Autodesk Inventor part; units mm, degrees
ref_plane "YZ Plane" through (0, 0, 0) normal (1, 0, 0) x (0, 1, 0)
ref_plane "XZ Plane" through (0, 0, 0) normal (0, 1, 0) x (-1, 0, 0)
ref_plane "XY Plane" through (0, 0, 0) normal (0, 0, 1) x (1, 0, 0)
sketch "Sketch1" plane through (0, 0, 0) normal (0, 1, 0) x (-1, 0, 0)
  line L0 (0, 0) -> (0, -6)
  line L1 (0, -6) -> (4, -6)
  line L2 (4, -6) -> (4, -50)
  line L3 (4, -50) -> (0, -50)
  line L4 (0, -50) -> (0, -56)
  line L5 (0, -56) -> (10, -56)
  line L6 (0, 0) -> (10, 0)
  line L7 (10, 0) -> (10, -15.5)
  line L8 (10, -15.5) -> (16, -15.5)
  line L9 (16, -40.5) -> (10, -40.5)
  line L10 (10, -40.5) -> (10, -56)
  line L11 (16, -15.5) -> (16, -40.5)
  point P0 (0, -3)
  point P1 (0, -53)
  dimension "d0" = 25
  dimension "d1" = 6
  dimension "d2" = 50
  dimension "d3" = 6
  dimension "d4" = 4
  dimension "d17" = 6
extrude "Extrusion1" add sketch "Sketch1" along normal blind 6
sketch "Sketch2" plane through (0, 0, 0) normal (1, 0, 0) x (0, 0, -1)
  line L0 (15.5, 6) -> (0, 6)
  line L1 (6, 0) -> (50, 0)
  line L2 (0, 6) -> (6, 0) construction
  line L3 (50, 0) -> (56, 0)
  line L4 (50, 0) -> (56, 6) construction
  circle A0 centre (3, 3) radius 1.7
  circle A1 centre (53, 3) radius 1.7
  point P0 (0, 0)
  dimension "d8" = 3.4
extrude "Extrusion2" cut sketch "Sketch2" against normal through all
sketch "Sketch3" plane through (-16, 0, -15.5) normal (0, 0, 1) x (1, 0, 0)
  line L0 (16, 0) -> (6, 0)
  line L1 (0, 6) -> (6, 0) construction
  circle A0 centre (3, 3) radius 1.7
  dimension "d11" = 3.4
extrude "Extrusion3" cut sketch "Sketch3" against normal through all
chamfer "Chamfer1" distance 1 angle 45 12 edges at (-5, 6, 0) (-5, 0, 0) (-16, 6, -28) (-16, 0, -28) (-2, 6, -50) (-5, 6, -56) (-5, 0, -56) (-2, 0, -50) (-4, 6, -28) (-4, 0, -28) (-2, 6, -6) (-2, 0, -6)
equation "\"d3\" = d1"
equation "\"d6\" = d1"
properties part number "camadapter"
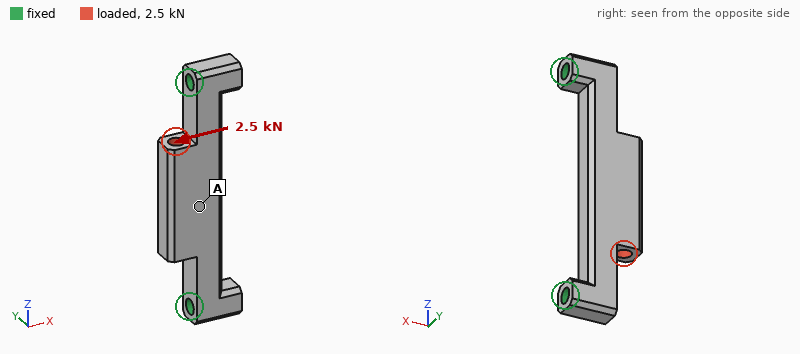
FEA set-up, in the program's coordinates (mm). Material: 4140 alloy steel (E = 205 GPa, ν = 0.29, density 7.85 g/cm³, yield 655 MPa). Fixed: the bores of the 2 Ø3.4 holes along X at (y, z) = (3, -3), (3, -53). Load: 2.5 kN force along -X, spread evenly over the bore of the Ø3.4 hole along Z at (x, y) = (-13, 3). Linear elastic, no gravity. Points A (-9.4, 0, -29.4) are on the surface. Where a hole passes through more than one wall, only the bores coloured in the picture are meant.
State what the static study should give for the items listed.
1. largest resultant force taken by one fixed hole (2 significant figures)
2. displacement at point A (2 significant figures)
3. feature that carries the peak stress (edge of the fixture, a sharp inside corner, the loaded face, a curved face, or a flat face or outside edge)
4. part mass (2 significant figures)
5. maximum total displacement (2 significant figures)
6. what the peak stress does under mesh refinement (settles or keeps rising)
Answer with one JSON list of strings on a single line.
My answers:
["1.5 kN", "28 µm", "edge of the fixture", "21 g", "28 µm", "keeps rising"]
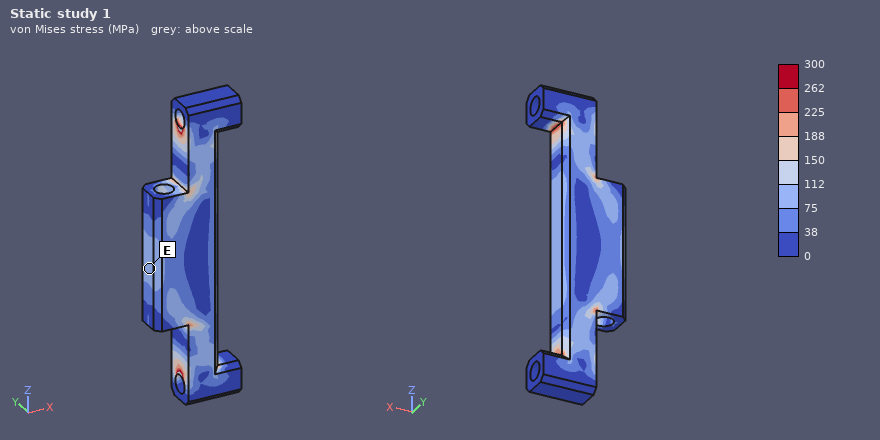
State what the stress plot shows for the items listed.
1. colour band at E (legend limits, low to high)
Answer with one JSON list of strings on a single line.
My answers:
["75 to 112 MPa"]
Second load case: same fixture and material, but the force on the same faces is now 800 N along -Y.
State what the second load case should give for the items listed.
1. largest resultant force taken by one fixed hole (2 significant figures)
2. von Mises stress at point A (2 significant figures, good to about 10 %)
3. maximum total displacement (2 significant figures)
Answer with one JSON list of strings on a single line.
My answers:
["400 N", "55 MPa", "39 µm"]
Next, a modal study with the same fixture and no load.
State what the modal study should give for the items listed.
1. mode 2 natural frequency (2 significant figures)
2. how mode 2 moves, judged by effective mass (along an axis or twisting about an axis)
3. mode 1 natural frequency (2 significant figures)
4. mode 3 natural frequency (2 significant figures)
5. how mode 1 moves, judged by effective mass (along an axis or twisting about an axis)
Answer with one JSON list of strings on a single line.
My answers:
["14 kHz", "along X", "9300 Hz", "18 kHz", "along Y"]
